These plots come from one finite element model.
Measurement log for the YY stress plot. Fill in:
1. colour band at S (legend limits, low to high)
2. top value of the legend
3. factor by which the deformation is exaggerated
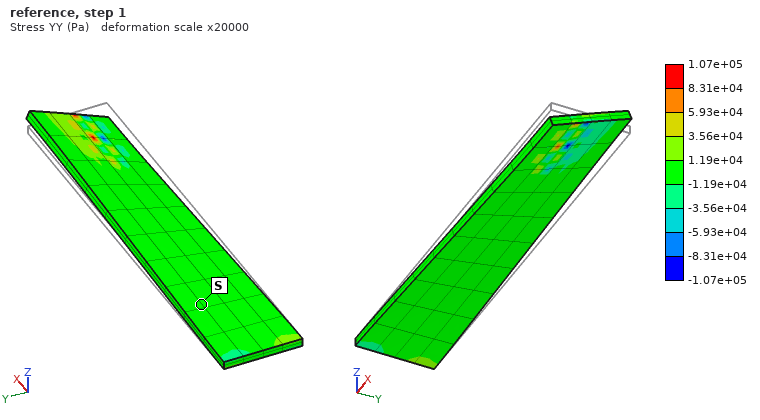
-1.19e+04 to 1.19e+04 Pa
1.07e+05 Pa
20000
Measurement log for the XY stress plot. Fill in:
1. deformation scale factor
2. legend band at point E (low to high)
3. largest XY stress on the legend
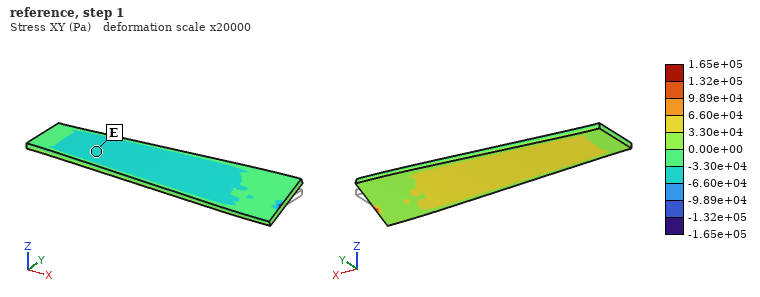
20000
-6.60e+04 to -3.30e+04 Pa
1.65e+05 Pa
